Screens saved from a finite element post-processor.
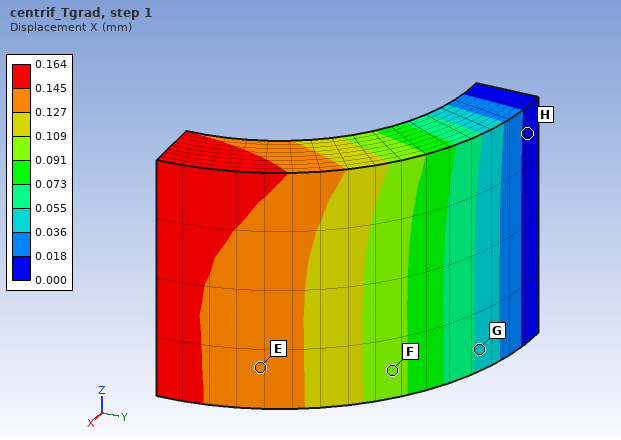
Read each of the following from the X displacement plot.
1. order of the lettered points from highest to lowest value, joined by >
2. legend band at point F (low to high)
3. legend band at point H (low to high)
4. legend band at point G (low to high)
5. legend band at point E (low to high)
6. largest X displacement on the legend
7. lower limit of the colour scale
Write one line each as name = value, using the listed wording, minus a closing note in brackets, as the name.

order of the lettered points from highest to lowest value, joined by > = E > F > G > H
legend band at point F = 0.091 to 0.109 mm
legend band at point H = 0.000 to 0.018 mm
legend band at point G = 0.036 to 0.055 mm
legend band at point E = 0.127 to 0.145 mm
largest X displacement on the legend = 0.164 mm
lower limit of the colour scale = 0.000 mm
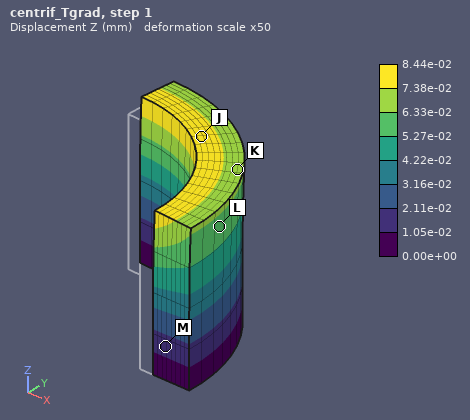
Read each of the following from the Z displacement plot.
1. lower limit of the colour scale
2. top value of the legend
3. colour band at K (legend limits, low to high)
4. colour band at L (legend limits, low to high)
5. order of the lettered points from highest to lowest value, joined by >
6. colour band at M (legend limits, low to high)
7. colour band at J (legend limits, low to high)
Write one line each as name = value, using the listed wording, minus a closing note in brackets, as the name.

lower limit of the colour scale = 0.00e+00 mm
top value of the legend = 8.44e-02 mm
colour band at K = 6.33e-02 to 7.38e-02 mm
colour band at L = 5.27e-02 to 6.33e-02 mm
order of the lettered points from highest to lowest value, joined by > = J > K > L > M
colour band at M = 1.05e-02 to 2.11e-02 mm
colour band at J = 7.38e-02 to 8.44e-02 mm
